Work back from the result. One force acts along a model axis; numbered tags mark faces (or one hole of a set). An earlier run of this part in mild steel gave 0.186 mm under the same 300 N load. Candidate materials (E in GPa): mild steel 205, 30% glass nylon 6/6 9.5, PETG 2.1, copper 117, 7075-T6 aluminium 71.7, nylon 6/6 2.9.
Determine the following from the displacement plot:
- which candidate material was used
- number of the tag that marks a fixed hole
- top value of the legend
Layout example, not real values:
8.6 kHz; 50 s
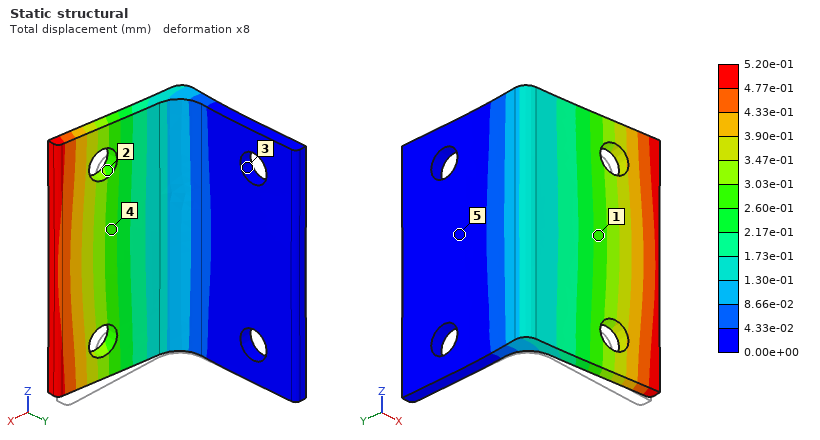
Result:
7075-T6 aluminium; 3; 5.20e-01 mm
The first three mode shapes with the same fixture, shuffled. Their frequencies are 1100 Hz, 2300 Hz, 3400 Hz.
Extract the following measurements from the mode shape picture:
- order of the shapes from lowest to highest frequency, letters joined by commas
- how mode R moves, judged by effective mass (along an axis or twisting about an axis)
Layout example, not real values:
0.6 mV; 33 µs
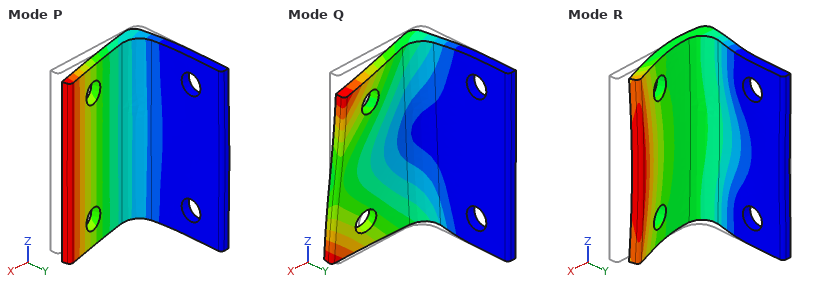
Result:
P, Q, R; along X
